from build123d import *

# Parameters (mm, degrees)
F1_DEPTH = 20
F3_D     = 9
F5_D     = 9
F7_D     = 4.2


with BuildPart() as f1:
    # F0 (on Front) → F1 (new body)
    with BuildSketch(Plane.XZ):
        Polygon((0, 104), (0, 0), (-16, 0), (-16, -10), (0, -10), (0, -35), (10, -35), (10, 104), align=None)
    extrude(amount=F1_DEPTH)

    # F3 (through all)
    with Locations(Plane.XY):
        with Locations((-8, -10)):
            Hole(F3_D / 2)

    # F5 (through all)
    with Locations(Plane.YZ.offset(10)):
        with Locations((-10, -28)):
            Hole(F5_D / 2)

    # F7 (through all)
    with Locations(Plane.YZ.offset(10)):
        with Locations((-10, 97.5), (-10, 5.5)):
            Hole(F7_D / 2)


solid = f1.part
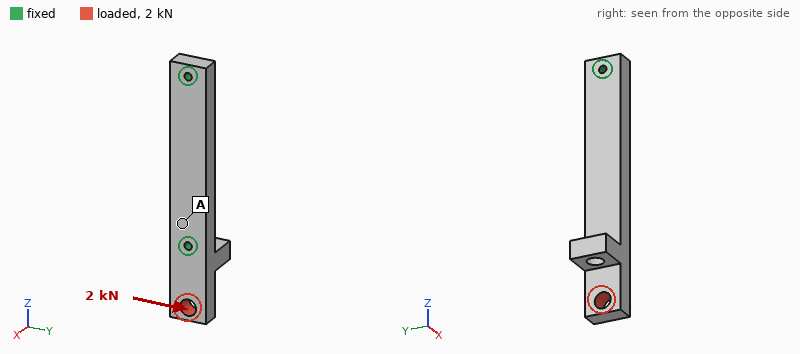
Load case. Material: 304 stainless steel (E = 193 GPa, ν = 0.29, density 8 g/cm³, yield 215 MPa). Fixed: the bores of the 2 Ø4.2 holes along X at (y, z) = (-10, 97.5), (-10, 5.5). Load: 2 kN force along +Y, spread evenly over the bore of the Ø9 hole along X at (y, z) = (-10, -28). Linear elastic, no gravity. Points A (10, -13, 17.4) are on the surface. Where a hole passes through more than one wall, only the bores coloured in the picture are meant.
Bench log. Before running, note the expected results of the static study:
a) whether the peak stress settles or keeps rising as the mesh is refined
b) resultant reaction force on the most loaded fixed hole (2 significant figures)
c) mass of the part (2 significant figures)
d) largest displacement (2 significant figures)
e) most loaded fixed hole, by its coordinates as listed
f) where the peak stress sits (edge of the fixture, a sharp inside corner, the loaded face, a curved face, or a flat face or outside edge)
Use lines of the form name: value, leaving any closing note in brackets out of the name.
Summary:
whether the peak stress settles or keeps rising as the mesh is refined: keeps rising
resultant reaction force on the most loaded fixed hole: 2.4 kN
mass of the part: 240 g
largest displacement: 65 µm
most loaded fixed hole, by its coordinates as listed: (-10, 5.5)
where the peak stress sits: edge of the fixture
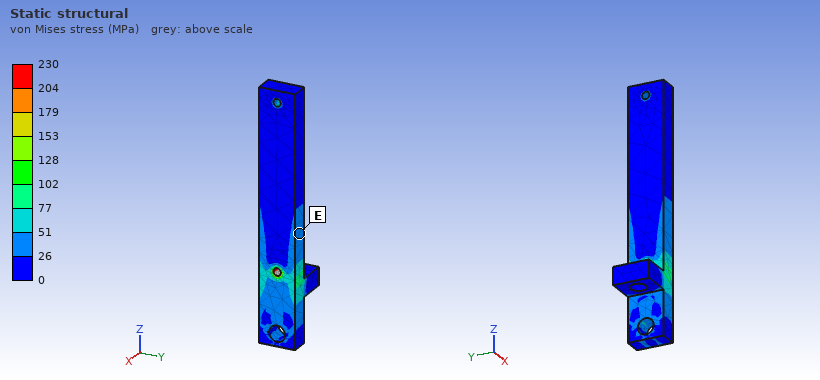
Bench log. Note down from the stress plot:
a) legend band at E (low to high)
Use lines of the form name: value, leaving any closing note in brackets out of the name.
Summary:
legend band at E: 26 to 51 MPa
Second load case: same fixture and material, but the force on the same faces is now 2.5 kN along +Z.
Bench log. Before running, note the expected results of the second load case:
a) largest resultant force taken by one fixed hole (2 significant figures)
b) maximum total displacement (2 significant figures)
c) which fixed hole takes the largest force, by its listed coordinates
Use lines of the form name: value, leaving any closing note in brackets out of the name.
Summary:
largest resultant force taken by one fixed hole: 2.4 kN
maximum total displacement: 4.5 µm
which fixed hole takes the largest force, by its listed coordinates: (-10, 5.5)
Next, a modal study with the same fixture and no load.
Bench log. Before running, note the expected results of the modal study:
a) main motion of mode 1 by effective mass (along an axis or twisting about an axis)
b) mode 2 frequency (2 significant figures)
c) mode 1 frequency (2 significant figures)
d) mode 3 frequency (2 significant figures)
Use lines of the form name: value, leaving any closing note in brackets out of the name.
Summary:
main motion of mode 1 by effective mass: twisting about Y
mode 2 frequency: 5400 Hz
mode 1 frequency: 4700 Hz
mode 3 frequency: 5500 Hz
